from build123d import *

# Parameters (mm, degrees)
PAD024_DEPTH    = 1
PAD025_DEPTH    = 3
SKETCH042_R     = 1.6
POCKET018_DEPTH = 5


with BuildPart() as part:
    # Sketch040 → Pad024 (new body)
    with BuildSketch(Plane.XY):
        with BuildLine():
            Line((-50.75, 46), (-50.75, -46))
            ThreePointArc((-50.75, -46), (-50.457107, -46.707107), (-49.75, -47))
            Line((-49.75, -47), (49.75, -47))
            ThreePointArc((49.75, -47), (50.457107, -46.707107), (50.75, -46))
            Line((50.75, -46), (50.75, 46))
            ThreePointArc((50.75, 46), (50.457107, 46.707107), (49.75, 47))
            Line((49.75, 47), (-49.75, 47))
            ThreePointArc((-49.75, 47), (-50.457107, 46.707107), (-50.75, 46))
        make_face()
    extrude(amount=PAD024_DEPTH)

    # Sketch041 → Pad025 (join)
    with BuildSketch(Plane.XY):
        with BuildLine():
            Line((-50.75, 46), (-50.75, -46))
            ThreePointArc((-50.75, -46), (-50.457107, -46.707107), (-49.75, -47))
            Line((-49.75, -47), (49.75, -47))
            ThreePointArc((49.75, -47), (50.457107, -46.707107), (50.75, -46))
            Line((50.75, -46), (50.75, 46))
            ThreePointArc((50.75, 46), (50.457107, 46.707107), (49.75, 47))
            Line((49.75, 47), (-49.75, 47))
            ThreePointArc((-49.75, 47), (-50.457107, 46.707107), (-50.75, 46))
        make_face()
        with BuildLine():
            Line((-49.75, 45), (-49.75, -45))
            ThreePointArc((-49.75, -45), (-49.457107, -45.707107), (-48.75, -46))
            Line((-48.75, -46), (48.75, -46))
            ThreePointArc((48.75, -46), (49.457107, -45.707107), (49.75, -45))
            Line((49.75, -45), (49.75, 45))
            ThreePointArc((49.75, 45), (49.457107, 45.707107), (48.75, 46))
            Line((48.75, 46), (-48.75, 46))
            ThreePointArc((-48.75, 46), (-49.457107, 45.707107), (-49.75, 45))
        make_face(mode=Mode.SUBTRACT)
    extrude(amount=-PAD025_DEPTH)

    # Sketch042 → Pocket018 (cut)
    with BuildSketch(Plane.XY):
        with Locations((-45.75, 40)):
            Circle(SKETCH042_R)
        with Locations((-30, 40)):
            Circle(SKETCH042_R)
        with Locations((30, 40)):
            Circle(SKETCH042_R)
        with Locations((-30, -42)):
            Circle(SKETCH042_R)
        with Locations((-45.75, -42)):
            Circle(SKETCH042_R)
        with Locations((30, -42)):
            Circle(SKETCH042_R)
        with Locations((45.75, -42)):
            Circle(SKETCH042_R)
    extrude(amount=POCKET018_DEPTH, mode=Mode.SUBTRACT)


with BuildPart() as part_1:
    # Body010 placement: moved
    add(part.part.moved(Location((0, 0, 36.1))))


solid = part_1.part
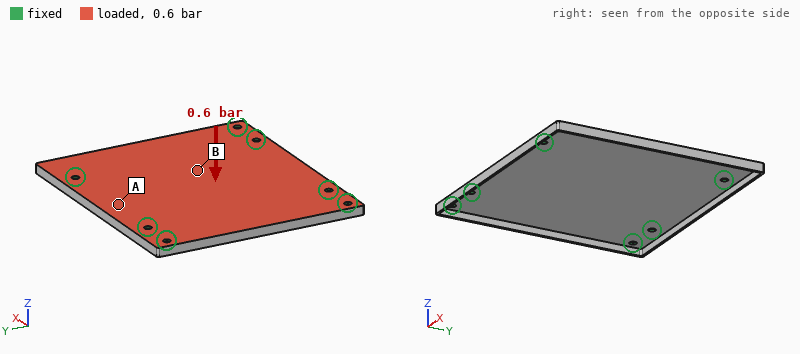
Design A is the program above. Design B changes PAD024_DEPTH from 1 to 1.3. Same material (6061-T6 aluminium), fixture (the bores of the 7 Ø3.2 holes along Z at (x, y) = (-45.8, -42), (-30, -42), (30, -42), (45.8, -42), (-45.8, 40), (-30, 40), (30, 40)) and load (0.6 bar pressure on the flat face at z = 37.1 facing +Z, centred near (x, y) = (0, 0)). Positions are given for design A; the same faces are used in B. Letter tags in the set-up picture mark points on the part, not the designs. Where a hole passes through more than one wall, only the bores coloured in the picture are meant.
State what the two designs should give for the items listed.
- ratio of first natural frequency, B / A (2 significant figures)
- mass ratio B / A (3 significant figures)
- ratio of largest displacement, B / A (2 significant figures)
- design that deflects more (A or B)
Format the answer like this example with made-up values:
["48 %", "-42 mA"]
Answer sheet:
["1.3", "1.27", "0.47", "A"]
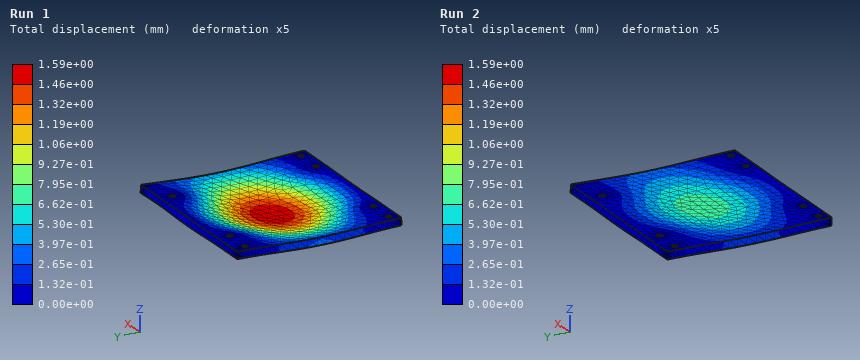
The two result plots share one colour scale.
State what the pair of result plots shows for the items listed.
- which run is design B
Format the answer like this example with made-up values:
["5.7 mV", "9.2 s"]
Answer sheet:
["Run 2"]
